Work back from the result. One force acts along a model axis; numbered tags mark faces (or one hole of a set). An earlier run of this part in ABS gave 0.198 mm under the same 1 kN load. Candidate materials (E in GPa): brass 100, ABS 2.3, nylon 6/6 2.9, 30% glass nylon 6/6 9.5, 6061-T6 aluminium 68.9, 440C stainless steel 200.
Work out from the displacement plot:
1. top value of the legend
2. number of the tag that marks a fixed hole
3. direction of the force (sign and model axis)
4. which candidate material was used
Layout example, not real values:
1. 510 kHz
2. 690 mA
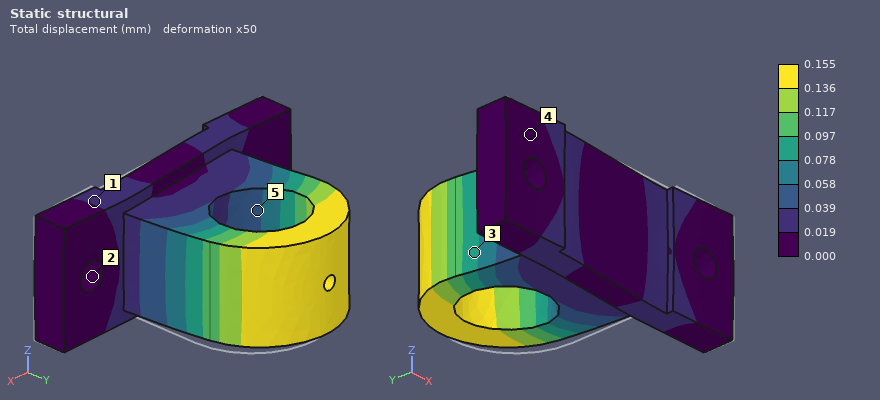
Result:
1. 0.155 mm
2. 2
3. -X
4. nylon 6/6
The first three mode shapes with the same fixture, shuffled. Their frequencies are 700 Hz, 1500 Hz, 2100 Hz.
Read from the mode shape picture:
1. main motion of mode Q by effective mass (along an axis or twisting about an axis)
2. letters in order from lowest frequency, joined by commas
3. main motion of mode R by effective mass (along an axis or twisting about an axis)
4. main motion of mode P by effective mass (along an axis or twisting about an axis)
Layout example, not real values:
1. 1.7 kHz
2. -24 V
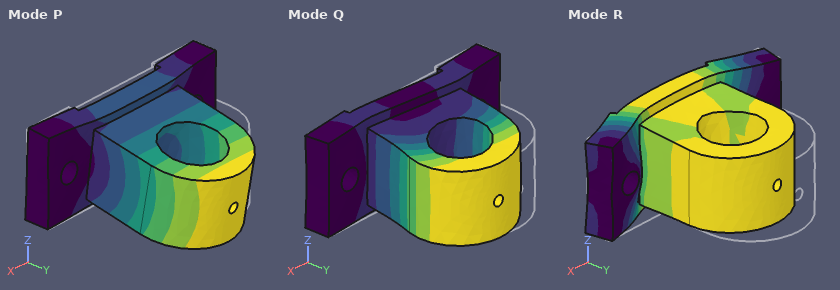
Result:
1. along X
2. P, Q, R
3. along Y
4. along Z
